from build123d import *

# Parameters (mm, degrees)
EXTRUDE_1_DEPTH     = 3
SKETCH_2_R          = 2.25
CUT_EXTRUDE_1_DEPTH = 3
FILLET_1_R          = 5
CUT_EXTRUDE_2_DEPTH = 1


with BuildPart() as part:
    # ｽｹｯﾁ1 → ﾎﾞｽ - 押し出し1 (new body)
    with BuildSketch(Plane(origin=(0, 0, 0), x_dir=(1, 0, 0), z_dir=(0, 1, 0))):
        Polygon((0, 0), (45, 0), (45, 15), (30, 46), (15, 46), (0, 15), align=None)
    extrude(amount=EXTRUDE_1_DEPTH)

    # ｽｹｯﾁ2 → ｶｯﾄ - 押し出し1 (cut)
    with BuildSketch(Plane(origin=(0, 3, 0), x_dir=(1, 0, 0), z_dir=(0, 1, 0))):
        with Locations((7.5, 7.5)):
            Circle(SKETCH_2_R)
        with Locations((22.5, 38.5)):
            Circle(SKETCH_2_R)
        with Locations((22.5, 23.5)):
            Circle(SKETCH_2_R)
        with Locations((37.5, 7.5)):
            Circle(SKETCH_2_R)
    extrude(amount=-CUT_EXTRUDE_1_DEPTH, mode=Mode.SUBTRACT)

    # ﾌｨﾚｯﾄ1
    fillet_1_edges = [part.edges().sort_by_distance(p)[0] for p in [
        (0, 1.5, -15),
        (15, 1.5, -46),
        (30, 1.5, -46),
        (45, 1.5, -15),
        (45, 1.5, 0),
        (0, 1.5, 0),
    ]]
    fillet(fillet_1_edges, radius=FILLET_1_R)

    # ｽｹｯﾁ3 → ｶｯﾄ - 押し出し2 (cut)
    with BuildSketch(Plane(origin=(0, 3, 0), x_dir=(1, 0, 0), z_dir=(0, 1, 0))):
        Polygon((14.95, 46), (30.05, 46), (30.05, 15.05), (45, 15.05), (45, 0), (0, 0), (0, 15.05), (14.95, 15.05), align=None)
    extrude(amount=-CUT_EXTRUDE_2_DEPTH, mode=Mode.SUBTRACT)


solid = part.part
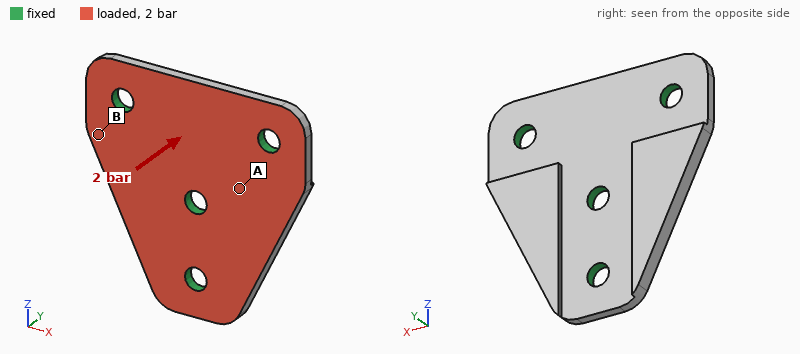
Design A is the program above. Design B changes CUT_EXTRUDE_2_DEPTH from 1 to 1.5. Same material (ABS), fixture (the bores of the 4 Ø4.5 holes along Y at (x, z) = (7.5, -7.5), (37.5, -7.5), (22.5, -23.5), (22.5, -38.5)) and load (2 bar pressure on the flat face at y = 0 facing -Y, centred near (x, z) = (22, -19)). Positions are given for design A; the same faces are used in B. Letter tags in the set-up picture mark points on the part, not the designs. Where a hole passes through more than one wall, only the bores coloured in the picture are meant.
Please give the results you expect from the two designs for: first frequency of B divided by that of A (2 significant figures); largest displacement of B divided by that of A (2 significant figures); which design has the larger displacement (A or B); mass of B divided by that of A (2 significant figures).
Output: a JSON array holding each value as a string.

["0.76", "1.9", "B", "0.85"]
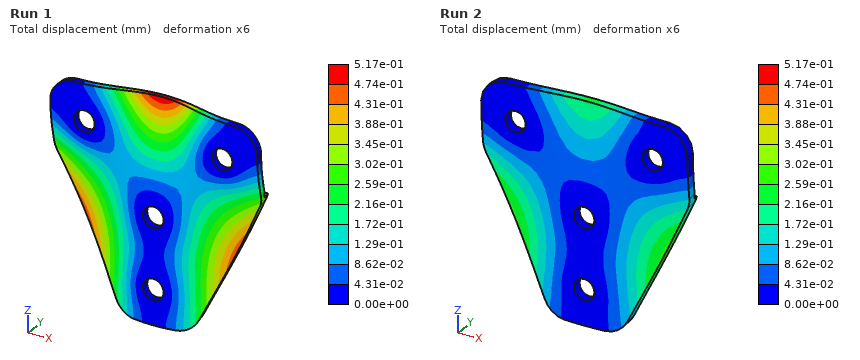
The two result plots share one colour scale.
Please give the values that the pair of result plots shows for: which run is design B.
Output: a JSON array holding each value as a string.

["Run 1"]
